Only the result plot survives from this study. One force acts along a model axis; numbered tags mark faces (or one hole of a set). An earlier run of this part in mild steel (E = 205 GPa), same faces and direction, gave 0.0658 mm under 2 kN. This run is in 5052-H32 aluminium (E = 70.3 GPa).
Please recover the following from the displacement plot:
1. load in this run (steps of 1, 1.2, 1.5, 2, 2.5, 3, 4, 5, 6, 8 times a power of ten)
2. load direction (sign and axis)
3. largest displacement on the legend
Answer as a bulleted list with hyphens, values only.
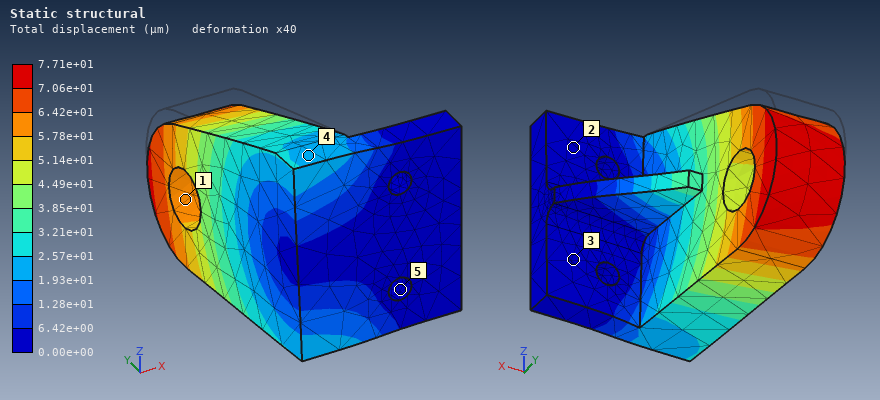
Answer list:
- 800 N
- -Z
- 7.71e+01 µm
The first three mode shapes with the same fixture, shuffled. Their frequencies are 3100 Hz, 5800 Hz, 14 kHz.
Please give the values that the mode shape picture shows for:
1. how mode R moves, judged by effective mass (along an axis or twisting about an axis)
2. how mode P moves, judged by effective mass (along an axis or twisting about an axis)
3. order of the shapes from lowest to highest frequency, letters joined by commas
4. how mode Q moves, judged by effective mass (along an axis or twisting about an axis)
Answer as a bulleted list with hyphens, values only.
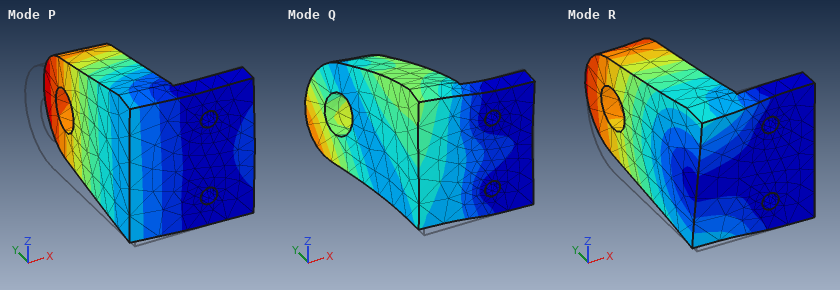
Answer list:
- along Z
- along X
- P, R, Q
- along Y
